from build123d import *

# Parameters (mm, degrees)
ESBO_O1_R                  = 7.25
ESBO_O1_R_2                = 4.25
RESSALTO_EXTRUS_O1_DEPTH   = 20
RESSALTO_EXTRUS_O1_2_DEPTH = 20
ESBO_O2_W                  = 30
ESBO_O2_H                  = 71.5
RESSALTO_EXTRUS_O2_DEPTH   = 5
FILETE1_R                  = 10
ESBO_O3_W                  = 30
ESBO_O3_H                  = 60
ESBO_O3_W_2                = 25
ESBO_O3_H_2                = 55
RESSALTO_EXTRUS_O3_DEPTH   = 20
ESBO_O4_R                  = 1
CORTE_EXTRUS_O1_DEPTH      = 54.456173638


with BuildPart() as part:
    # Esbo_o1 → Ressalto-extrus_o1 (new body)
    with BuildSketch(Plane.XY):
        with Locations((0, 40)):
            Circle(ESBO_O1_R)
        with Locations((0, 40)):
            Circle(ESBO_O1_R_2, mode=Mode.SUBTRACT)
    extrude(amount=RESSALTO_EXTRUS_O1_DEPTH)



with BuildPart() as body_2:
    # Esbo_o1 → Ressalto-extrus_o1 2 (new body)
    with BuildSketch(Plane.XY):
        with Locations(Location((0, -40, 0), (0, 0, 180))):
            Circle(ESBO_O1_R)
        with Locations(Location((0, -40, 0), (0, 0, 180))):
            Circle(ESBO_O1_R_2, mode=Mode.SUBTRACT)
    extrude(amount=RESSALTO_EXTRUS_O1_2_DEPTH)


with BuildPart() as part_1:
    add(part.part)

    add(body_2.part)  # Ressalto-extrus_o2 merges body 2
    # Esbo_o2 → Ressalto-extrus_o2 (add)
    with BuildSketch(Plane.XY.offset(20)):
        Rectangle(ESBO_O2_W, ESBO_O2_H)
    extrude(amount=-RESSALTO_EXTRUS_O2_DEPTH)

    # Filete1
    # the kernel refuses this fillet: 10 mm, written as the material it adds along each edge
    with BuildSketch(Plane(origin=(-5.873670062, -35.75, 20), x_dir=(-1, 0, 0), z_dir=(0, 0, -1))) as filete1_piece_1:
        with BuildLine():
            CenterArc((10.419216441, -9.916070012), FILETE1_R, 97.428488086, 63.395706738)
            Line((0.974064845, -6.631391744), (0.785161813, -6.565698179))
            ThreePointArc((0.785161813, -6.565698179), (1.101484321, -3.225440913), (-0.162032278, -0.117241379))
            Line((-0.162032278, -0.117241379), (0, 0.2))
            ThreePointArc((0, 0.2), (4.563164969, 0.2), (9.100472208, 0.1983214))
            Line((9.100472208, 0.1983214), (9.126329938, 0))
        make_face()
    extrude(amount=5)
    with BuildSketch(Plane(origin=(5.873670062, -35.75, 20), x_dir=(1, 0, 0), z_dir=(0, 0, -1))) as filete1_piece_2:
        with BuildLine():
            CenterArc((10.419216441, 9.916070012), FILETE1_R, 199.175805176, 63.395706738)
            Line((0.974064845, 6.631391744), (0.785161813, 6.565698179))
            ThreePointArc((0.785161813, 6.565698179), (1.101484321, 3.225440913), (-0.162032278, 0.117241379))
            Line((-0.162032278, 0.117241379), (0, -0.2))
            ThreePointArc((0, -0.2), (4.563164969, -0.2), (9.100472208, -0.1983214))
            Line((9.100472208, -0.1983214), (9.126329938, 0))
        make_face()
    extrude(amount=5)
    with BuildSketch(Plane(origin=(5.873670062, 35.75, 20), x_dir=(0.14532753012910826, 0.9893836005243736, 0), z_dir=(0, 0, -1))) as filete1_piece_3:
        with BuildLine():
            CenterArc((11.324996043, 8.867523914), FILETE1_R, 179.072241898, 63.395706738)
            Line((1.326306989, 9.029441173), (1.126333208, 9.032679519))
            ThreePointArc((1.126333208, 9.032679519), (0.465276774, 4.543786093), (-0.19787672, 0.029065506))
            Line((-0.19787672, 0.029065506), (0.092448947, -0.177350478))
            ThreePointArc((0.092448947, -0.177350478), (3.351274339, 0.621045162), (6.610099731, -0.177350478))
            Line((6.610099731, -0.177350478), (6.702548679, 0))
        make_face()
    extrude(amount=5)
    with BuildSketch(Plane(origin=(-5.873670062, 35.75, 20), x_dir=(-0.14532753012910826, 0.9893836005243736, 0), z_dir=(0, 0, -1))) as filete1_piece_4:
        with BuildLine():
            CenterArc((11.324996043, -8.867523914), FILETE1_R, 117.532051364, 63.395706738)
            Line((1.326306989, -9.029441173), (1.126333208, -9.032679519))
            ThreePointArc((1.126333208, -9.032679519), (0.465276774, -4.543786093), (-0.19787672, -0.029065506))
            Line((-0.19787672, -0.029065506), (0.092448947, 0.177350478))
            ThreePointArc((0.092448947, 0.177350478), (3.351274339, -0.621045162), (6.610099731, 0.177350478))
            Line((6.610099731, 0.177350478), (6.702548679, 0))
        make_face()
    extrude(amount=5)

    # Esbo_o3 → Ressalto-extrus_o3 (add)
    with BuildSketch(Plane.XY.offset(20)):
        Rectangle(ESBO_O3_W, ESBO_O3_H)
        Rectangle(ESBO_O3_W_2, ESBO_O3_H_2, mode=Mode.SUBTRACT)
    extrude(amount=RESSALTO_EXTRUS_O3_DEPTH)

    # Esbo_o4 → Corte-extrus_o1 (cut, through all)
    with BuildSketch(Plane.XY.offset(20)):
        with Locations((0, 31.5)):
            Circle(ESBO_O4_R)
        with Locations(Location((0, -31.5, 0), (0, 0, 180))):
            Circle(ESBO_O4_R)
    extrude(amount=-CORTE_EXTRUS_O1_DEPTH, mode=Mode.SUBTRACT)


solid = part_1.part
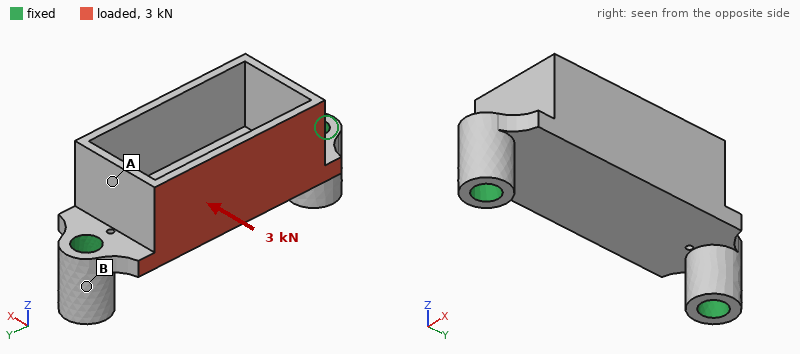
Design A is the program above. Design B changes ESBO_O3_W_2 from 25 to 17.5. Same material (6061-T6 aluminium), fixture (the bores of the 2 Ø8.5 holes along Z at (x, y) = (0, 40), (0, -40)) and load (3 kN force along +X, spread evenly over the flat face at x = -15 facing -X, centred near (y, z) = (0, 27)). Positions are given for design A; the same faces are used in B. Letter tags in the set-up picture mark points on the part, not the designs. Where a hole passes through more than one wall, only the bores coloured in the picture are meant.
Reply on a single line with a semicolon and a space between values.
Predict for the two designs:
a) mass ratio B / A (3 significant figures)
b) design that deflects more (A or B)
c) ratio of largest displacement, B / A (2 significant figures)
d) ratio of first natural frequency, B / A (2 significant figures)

1.35; A; 0.35; 0.84
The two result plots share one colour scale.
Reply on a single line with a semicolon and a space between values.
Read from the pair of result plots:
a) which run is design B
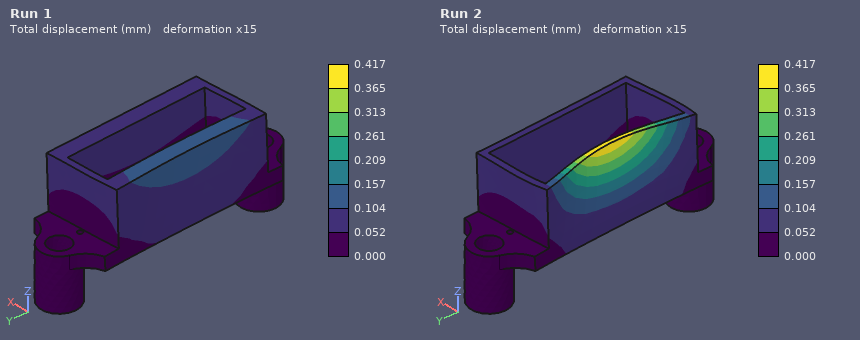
Run 1
